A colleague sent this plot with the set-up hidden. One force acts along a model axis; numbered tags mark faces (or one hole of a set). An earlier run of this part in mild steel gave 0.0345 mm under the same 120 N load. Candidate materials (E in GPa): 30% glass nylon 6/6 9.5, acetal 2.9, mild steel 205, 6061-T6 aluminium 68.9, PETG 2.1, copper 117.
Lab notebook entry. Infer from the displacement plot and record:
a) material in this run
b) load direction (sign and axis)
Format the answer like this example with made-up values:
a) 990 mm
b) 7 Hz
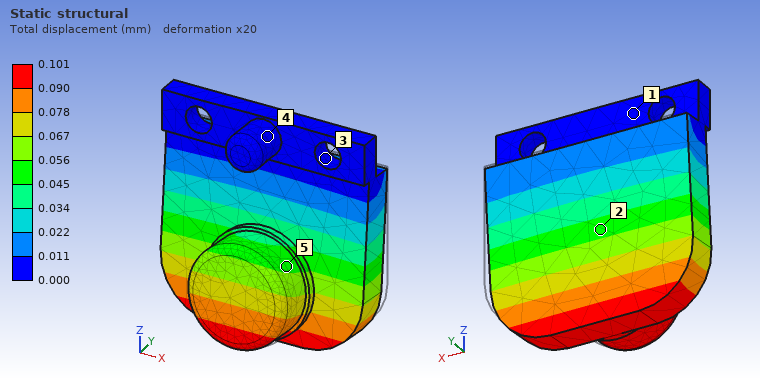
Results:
a) 6061-T6 aluminium
b) -Y
